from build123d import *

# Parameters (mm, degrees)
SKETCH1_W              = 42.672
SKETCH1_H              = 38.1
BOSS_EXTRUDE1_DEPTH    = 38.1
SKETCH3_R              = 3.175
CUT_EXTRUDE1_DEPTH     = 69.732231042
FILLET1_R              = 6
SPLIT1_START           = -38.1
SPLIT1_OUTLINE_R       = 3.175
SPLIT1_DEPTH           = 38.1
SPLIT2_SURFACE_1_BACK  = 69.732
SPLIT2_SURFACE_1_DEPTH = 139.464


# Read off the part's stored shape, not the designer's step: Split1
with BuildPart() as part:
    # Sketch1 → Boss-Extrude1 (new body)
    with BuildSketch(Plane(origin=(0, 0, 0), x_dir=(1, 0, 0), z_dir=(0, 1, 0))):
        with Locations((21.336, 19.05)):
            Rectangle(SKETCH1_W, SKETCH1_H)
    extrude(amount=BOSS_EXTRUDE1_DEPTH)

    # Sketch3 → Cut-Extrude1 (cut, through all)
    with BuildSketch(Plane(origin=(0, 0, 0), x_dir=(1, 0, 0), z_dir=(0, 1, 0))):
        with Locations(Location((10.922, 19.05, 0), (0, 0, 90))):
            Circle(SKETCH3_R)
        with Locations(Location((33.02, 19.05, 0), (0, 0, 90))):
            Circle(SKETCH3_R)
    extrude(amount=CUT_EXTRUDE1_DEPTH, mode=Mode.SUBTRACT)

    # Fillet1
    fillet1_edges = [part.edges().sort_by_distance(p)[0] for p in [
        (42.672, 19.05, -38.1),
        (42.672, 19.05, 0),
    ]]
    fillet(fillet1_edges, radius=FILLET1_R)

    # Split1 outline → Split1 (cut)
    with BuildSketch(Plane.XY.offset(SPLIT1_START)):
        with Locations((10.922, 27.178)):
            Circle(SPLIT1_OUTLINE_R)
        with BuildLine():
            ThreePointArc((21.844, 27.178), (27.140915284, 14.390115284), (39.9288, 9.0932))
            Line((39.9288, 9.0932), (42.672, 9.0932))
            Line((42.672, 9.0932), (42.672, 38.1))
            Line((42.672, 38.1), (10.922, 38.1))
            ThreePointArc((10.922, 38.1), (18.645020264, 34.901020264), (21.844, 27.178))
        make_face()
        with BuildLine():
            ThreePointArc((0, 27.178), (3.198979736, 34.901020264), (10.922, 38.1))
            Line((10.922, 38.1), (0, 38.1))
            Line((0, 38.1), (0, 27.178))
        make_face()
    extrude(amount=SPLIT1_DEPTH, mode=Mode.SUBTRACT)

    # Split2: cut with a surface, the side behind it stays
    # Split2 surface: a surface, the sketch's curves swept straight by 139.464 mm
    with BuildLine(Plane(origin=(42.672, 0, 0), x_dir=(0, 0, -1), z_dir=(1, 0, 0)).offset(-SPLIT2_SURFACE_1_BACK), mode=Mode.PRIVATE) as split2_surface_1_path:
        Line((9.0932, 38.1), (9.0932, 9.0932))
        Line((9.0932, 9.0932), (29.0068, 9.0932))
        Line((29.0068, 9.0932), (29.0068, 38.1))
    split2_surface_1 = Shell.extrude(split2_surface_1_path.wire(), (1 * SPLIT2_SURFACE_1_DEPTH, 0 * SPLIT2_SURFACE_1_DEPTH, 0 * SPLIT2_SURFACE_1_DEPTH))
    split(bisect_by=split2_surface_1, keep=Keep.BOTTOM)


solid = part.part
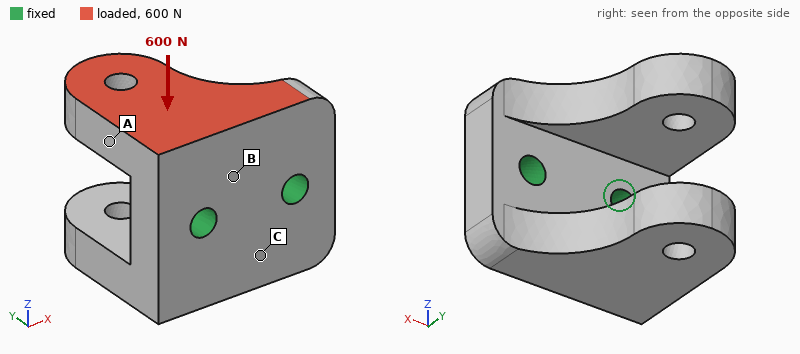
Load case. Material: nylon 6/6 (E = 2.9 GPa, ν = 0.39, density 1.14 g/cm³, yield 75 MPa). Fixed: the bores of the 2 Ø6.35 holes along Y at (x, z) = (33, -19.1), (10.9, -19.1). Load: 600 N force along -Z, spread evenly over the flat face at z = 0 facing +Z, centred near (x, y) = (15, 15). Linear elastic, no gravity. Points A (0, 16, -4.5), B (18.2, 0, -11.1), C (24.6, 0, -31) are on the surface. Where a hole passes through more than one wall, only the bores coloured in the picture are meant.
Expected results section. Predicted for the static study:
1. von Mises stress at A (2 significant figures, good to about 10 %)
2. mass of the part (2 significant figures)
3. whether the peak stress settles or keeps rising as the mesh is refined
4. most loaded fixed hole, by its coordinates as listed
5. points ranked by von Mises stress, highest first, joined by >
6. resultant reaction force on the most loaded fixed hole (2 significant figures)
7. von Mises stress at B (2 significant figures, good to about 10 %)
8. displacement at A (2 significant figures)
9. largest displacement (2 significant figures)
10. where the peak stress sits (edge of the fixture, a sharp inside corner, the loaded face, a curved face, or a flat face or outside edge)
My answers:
4.1 MPa
29 g
keeps rising
(10.9, -19.1)
B > A > C
480 N
9.0 MPa
0.23 mm
0.73 mm
edge of the fixture
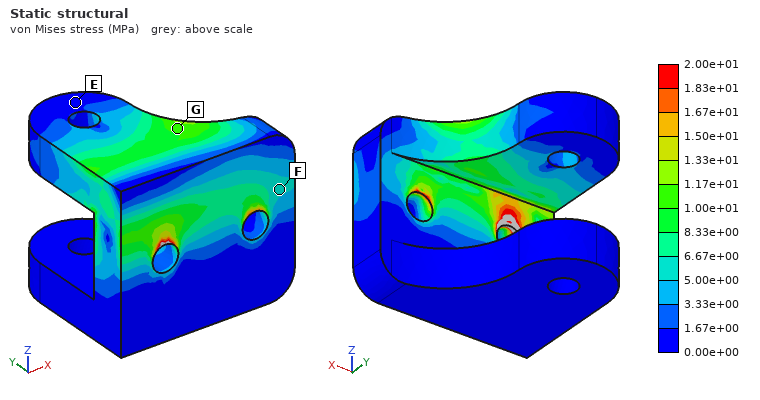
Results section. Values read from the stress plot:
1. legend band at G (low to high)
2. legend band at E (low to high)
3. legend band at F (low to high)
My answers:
1.00e+01 to 1.17e+01 MPa
0.00e+00 to 1.67e+00 MPa
5.00e+00 to 6.67e+00 MPa
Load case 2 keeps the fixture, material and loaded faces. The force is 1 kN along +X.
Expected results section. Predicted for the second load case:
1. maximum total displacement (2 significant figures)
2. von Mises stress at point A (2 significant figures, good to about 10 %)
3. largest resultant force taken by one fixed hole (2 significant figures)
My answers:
0.35 mm
5.6 MPa
940 N
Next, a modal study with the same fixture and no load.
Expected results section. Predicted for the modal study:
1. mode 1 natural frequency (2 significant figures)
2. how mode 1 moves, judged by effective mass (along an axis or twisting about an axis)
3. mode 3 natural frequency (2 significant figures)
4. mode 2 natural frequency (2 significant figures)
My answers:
1700 Hz
along Z
3100 Hz
1800 Hz
